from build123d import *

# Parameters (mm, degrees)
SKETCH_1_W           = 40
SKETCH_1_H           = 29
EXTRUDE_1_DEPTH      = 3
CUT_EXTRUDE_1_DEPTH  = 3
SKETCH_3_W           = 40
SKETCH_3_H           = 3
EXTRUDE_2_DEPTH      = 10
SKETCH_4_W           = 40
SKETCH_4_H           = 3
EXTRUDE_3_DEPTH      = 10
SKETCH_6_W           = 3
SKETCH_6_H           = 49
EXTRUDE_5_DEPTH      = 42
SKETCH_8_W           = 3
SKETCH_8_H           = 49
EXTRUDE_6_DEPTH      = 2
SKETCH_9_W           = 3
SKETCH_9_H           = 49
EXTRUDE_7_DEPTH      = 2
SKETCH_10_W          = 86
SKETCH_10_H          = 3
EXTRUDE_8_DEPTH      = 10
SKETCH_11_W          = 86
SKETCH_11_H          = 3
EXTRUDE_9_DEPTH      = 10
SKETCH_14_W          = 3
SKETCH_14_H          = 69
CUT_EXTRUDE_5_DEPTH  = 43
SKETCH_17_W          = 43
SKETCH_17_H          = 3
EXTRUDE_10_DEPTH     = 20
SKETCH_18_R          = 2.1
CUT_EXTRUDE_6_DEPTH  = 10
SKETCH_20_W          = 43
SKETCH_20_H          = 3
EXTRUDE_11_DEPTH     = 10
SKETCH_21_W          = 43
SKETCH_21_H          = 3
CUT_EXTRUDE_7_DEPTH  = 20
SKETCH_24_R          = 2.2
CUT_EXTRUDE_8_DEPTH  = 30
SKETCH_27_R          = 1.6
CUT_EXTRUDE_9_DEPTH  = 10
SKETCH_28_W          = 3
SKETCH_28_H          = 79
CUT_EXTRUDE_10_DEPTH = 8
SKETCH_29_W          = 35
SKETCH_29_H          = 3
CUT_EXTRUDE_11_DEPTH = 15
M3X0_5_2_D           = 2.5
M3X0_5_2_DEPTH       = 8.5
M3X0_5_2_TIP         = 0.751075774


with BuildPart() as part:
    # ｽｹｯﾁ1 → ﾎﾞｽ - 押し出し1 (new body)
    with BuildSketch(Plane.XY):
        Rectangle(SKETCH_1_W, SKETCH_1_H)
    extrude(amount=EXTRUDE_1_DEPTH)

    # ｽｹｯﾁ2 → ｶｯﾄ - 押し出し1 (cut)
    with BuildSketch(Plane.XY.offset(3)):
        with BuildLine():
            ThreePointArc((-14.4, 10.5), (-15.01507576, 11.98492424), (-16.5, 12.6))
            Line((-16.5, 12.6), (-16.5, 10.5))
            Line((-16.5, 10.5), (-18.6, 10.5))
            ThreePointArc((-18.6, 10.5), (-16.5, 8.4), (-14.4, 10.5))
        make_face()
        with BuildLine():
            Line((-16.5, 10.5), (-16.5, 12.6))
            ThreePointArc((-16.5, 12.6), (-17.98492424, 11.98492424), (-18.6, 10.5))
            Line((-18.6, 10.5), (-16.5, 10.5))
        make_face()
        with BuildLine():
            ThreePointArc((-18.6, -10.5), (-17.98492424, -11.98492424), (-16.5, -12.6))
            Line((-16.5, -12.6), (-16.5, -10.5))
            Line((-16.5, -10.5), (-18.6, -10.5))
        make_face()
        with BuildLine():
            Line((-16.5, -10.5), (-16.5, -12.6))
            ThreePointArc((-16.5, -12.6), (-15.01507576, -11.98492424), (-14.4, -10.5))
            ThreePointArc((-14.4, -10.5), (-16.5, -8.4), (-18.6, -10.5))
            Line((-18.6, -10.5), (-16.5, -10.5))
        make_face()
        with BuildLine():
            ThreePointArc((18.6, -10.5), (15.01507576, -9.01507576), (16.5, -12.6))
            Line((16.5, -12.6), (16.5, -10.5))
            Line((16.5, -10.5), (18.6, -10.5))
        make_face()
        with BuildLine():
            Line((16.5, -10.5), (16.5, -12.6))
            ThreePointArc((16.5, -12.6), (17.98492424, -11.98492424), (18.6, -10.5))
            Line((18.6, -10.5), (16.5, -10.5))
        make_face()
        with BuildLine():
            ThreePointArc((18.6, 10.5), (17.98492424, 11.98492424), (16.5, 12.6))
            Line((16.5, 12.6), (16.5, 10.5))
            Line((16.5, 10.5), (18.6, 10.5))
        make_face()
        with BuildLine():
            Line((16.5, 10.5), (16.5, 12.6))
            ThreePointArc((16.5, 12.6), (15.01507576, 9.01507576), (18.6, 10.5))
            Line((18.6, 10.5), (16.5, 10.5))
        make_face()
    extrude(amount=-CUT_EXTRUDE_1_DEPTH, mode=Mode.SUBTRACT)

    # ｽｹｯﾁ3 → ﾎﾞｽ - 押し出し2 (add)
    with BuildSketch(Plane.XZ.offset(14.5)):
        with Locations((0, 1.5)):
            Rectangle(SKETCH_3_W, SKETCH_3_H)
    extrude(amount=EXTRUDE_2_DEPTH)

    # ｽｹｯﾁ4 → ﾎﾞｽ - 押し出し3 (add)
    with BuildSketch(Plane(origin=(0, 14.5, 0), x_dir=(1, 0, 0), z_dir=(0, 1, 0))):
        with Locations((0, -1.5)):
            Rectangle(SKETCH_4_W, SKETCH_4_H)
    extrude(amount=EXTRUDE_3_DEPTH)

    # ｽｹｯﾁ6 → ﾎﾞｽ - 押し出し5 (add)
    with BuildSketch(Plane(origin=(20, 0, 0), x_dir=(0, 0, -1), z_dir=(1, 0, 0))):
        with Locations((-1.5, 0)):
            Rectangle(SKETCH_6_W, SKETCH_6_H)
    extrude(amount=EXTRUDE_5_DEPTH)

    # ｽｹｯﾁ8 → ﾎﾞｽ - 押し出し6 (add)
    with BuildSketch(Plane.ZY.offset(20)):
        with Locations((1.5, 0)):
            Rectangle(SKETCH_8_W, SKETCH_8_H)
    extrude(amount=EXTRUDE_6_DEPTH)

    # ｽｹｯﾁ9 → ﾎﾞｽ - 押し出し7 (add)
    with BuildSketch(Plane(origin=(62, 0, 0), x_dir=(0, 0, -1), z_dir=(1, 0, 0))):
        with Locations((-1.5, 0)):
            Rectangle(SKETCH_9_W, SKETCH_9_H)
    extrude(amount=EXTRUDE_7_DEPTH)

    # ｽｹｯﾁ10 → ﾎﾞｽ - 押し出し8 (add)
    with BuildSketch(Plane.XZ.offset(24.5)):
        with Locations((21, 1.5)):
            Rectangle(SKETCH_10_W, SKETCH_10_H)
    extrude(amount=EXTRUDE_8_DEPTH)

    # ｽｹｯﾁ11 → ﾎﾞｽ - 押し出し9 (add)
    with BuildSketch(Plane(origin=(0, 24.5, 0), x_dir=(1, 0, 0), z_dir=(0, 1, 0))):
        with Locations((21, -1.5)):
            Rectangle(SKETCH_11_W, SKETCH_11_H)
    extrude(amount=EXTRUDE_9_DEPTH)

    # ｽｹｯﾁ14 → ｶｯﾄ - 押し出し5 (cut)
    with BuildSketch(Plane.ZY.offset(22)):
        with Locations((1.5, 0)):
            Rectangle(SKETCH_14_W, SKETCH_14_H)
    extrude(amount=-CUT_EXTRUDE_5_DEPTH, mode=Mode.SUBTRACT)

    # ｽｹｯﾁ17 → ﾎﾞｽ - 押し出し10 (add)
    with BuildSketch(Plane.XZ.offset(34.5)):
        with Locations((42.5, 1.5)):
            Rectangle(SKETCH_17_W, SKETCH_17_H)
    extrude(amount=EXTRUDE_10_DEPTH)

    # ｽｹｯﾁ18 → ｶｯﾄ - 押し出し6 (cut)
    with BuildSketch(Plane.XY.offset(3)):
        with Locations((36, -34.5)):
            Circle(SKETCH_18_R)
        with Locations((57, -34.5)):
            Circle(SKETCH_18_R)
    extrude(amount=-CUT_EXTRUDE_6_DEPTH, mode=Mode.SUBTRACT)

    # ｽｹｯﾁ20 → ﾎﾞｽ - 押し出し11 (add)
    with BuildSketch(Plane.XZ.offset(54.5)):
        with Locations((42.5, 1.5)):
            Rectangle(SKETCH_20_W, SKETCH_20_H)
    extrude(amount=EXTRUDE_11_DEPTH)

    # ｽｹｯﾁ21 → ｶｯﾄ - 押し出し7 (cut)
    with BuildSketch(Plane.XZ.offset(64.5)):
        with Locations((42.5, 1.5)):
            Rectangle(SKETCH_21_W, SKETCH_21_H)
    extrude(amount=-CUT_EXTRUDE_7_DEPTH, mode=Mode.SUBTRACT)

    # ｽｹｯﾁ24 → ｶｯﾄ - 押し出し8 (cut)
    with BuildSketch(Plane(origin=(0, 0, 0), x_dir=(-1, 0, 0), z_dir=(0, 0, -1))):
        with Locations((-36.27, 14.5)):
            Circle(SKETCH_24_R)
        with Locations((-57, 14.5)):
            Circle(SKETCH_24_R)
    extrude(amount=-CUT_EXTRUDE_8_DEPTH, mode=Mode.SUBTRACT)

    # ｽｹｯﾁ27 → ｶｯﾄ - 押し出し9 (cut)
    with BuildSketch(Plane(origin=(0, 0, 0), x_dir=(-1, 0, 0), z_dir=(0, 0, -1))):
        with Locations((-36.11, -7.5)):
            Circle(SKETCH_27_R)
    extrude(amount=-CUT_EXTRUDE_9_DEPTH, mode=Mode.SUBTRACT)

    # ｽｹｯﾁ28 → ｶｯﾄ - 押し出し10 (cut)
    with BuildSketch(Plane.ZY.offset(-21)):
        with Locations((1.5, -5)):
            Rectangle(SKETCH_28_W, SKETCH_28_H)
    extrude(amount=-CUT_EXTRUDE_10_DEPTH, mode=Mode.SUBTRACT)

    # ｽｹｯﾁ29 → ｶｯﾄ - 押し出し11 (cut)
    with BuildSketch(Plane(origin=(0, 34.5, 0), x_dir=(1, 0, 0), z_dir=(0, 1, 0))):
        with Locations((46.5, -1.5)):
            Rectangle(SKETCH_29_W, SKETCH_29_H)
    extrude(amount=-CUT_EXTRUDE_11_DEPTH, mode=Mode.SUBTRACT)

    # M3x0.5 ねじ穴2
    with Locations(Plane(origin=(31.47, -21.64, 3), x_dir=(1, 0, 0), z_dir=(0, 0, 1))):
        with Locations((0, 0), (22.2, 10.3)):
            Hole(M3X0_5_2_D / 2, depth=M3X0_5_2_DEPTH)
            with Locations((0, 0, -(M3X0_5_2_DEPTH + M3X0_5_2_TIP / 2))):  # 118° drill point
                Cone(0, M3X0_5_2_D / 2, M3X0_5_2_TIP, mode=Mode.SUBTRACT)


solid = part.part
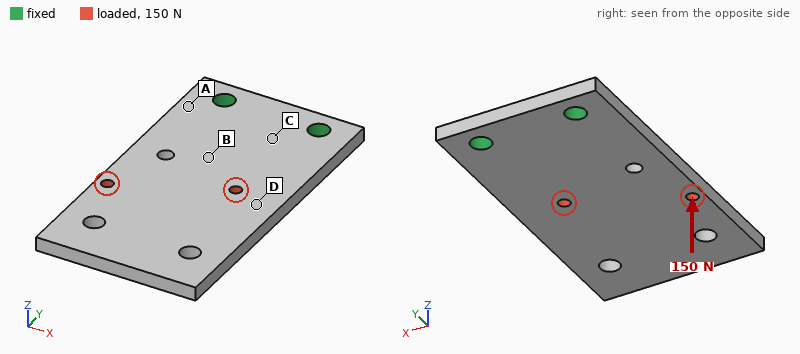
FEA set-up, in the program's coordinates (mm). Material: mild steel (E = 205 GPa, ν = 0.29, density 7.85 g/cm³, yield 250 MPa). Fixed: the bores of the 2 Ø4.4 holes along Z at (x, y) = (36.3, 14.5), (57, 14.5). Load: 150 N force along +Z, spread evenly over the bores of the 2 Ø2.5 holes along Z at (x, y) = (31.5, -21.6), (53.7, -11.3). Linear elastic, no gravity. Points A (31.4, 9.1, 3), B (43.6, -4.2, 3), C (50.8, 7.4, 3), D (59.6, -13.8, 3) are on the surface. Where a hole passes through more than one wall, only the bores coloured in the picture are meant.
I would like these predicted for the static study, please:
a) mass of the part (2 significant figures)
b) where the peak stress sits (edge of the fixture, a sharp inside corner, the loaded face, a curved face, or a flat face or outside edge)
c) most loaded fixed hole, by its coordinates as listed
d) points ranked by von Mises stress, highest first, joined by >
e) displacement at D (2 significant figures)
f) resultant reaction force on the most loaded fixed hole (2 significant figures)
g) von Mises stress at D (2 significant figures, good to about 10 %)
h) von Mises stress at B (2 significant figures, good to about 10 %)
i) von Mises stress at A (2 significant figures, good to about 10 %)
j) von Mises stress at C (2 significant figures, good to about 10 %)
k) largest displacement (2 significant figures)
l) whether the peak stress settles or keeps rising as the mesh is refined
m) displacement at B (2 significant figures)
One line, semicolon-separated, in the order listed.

51 g; edge of the fixture; (36.3, 14.5); A > C > B > D; 0.067 mm; 99 N; 13 MPa; 35 MPa; 77 MPa; 57 MPa; 0.22 mm; keeps rising; 0.039 mm
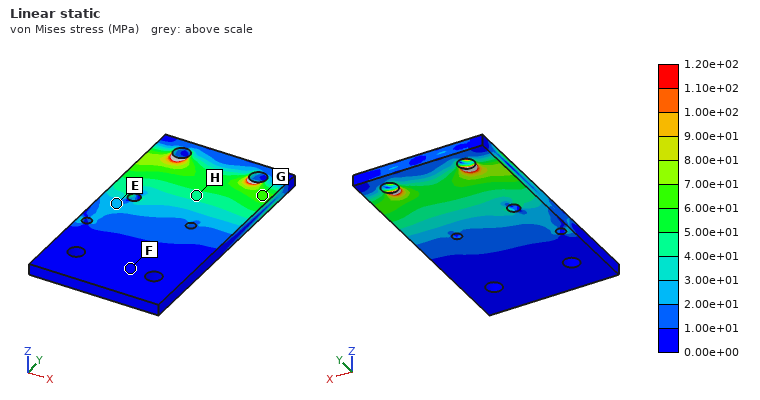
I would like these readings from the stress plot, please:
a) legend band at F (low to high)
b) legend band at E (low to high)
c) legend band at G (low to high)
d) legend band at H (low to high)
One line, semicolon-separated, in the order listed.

0.00e+00 to 1.00e+01 MPa; 2.00e+01 to 3.00e+01 MPa; 6.00e+01 to 7.00e+01 MPa; 4.00e+01 to 5.00e+01 MPa
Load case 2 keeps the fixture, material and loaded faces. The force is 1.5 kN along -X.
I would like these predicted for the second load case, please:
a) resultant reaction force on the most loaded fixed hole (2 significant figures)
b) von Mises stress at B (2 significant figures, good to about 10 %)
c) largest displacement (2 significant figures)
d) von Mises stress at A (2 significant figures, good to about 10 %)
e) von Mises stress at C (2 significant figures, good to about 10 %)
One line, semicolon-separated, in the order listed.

2.1 kN; 36 MPa; 27 µm; 43 MPa; 42 MPa
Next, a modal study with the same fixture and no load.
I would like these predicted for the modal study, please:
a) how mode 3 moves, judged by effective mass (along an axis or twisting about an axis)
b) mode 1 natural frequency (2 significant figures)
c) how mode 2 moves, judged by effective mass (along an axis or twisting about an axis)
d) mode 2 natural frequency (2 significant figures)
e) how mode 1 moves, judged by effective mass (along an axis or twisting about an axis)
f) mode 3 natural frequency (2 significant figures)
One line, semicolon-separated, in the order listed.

along Z; 740 Hz; twisting about Y; 2700 Hz; along Z; 4500 Hz
